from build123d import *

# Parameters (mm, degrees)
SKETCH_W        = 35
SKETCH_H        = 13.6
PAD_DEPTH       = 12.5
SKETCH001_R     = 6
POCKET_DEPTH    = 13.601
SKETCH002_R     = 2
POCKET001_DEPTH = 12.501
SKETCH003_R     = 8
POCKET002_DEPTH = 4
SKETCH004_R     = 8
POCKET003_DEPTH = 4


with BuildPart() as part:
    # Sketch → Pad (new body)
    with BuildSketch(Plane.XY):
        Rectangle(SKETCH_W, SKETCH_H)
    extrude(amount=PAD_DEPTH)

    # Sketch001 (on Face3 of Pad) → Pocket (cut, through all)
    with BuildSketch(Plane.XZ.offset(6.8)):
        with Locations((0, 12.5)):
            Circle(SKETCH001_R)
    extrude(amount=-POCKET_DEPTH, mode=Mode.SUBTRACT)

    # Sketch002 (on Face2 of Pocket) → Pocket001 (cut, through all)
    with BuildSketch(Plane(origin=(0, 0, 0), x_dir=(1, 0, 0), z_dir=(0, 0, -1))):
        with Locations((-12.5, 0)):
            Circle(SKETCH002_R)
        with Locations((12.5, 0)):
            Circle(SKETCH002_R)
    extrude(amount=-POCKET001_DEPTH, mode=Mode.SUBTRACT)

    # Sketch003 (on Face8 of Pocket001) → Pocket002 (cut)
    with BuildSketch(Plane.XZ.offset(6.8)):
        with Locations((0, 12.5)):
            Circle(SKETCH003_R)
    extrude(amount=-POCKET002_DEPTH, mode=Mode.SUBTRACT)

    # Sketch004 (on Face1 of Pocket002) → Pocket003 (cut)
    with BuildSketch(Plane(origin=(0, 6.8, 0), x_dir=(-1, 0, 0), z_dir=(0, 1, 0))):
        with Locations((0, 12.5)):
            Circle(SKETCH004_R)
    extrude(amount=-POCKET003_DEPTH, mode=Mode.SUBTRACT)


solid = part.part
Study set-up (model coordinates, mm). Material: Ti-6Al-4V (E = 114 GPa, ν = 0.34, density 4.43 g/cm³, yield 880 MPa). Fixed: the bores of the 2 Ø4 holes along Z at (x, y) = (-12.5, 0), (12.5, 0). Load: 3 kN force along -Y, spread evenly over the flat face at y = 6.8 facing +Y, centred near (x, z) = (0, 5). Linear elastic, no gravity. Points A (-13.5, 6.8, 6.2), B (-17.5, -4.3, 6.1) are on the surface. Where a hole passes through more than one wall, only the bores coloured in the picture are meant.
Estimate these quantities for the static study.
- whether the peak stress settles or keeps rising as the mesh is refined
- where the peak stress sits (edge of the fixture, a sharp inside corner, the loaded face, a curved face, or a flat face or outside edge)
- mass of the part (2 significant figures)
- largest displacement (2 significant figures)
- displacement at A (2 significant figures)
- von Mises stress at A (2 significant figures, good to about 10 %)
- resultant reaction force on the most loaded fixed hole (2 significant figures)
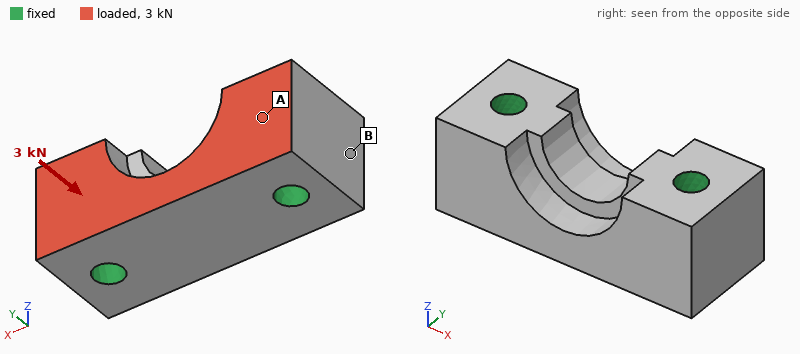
keeps rising
edge of the fixture
20 g
2.2 µm
0.49 µm
13 MPa
1.5 kN
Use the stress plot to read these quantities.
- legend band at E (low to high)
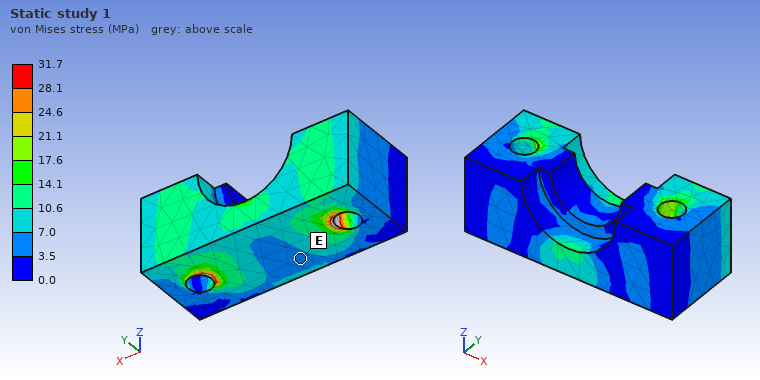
3.5 to 7.0 MPa
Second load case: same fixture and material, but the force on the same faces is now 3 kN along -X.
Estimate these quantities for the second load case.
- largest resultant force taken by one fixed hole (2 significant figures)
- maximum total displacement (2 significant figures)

1.6 kN
3.1 µm
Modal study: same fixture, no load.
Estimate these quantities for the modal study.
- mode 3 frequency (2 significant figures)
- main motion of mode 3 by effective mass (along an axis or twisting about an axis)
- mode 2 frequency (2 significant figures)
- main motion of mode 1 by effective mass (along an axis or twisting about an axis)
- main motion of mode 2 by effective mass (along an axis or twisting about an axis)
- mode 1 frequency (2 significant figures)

74 kHz
twisting about X
59 kHz
along Y
along Z
48 kHz
